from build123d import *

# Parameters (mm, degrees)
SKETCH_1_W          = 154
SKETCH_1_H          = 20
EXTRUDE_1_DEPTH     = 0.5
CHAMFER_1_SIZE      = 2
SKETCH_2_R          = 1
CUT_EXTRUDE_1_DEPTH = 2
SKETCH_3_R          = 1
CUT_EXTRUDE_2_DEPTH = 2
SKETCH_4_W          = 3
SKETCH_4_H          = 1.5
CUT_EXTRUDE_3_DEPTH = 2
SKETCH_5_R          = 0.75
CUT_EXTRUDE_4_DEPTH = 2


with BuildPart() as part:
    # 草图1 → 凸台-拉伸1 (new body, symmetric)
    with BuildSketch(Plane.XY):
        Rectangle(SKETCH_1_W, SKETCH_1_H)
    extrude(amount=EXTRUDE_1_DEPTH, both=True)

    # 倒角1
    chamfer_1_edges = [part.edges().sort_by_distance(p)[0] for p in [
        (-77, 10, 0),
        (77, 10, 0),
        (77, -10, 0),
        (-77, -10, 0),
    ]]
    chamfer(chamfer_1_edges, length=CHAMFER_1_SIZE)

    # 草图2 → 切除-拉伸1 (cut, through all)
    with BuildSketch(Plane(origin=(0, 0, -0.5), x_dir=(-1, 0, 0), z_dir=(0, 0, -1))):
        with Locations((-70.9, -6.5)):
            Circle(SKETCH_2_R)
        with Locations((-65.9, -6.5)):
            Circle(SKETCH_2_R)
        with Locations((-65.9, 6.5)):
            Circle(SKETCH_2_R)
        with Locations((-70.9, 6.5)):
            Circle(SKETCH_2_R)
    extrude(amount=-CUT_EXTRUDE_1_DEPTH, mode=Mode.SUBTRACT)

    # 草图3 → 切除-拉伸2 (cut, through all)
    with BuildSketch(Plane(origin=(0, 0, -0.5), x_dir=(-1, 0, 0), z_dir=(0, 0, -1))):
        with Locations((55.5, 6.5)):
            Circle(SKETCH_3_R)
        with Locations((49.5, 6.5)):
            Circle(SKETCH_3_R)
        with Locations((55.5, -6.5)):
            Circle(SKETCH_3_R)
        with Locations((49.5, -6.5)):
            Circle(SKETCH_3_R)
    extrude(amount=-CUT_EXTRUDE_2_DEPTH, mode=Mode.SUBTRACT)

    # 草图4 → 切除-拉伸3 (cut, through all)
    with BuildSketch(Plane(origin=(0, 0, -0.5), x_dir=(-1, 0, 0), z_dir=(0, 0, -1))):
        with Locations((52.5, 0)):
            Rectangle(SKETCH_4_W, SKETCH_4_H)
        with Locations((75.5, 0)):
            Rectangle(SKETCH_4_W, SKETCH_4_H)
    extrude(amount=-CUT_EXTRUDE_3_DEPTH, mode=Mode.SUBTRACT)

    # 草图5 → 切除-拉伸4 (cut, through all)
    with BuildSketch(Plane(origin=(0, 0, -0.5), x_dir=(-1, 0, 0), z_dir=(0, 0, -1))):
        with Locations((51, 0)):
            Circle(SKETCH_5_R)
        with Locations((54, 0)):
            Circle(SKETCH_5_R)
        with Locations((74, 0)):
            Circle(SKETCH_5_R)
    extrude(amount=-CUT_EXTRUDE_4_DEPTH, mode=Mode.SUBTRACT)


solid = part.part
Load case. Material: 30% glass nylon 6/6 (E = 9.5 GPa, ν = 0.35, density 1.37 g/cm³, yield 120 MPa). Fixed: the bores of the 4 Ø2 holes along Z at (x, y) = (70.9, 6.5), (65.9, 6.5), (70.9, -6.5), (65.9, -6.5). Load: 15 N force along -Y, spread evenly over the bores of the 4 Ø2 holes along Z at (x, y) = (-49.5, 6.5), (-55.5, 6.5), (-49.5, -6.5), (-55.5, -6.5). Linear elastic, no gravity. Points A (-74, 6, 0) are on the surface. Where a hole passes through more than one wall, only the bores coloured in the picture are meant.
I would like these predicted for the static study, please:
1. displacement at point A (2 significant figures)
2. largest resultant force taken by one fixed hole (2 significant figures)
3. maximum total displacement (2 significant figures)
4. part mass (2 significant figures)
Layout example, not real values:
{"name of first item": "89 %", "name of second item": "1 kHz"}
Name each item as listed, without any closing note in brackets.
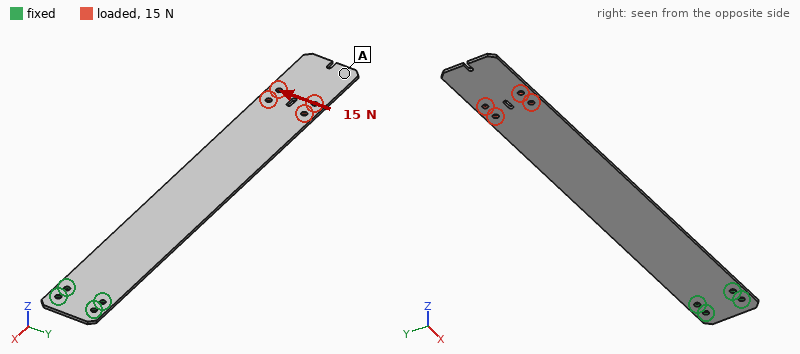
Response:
{"displacement at point A": "1.7 mm", "largest resultant force taken by one fixed hole": "110 N", "maximum total displacement": "1.8 mm", "part mass": "4.2 g"}
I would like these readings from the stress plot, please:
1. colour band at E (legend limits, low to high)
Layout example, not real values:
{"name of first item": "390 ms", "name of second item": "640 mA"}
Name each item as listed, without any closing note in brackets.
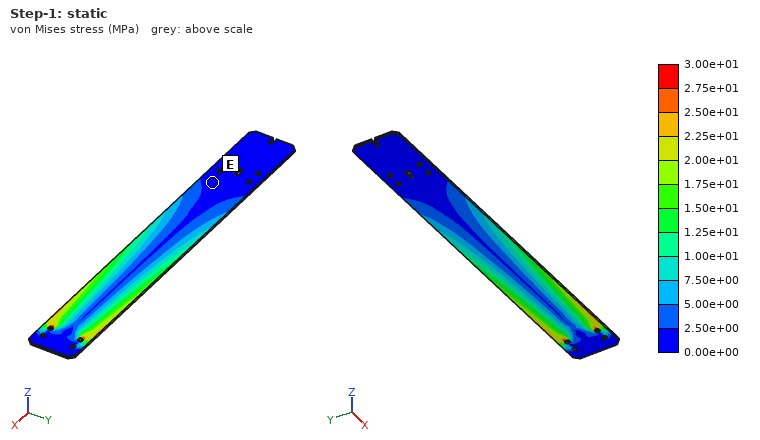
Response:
{"colour band at E": "0.00e+00 to 2.50e+00 MPa"}
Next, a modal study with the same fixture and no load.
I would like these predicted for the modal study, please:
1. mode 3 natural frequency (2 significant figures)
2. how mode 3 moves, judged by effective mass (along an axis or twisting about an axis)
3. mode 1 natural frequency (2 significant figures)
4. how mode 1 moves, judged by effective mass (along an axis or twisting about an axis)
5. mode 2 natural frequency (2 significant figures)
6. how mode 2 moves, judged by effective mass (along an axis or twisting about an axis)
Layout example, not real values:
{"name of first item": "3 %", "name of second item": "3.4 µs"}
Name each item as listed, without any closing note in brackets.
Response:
{"mode 3 natural frequency": "290 Hz", "how mode 3 moves, judged by effective mass": "twisting about X", "mode 1 natural frequency": "21 Hz", "how mode 1 moves, judged by effective mass": "along Z", "mode 2 natural frequency": "130 Hz", "how mode 2 moves, judged by effective mass": "along Z"}
